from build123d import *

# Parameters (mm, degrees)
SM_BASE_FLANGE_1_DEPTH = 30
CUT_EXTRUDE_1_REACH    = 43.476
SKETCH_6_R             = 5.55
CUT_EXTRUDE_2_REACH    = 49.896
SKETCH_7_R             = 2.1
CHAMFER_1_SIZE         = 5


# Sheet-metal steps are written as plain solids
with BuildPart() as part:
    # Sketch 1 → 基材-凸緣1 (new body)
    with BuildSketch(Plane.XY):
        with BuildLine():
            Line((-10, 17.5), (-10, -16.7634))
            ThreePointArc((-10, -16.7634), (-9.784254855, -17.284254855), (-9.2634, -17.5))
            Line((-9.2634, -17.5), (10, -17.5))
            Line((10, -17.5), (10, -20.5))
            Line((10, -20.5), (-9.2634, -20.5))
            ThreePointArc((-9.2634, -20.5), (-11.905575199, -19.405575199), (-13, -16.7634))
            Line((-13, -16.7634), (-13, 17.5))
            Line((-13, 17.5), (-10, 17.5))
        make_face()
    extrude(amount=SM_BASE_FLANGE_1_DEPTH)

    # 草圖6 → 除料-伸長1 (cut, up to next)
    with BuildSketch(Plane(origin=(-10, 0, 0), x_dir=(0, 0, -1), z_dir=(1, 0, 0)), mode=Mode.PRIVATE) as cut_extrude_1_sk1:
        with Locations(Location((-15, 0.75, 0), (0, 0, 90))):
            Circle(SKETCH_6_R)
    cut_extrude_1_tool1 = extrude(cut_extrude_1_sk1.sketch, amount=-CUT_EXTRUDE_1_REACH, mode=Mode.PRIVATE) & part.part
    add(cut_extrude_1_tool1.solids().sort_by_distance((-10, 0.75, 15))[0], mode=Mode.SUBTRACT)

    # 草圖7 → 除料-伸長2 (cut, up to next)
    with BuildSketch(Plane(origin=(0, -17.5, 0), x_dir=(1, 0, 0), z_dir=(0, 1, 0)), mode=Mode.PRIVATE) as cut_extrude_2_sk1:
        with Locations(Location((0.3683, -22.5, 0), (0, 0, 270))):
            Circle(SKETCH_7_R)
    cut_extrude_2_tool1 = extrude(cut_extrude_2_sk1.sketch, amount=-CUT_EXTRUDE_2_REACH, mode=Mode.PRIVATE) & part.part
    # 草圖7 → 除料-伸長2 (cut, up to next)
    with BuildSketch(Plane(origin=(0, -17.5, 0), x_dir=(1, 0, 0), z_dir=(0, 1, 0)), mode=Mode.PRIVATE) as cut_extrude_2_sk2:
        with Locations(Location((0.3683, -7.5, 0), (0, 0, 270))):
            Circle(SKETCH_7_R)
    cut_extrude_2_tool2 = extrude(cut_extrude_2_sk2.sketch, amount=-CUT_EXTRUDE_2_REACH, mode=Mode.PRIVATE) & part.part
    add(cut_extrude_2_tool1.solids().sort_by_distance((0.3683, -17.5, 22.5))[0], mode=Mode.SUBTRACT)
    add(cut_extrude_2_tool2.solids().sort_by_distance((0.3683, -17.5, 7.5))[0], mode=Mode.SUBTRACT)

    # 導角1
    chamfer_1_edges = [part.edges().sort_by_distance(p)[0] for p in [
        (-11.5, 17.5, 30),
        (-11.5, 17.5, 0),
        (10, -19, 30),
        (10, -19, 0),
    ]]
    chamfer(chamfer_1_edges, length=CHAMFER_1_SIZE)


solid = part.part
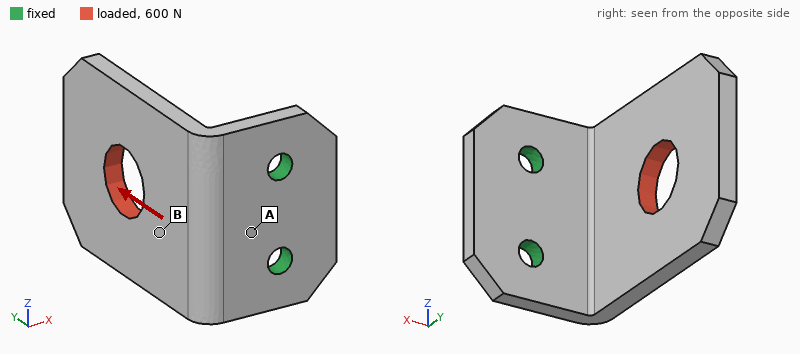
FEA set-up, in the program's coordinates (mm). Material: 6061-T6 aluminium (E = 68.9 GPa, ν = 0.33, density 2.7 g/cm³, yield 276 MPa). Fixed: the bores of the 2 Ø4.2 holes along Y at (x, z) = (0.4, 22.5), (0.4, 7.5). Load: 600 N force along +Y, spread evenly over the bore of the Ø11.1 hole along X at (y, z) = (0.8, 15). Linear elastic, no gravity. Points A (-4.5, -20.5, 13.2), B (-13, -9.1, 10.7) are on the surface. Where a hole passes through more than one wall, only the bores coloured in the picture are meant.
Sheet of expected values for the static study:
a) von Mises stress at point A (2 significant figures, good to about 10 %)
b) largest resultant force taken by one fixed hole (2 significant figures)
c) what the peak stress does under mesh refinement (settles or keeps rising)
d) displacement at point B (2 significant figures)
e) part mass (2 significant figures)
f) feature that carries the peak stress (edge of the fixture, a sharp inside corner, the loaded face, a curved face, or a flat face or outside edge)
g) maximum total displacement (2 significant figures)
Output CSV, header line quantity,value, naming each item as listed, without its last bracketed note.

quantity,value
von Mises stress at point A,73 MPa
largest resultant force taken by one fixed hole,300 N
what the peak stress does under mesh refinement,keeps rising
displacement at point B,0.10 mm
part mass,12 g
feature that carries the peak stress,edge of the fixture
maximum total displacement,0.29 mm
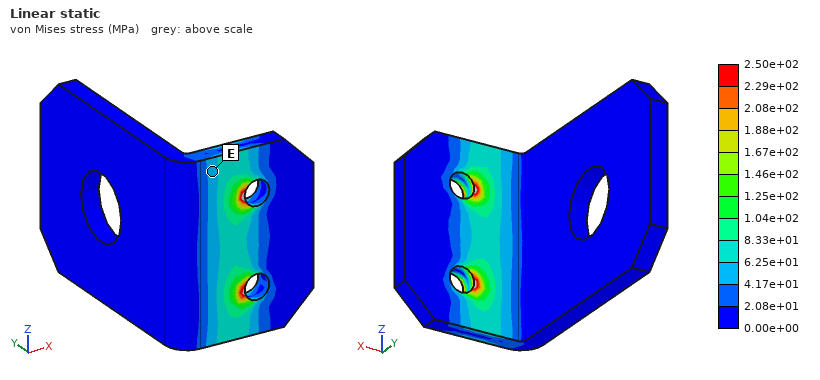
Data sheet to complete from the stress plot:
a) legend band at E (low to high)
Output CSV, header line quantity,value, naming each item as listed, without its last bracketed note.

quantity,value
legend band at E,4.17e+01 to 6.25e+01 MPa
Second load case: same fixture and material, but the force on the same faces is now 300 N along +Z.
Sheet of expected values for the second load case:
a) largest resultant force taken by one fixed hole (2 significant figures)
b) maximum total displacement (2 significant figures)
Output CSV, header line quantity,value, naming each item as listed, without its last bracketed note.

quantity,value
largest resultant force taken by one fixed hole,390 N
maximum total displacement,0.14 mm
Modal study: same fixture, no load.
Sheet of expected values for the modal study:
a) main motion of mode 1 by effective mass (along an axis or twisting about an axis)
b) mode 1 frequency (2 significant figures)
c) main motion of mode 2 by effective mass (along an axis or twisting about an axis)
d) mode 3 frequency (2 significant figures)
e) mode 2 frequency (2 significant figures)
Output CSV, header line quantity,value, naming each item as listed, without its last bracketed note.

quantity,value
main motion of mode 1 by effective mass,along X
mode 1 frequency,1400 Hz
main motion of mode 2 by effective mass,along Z
mode 3 frequency,5000 Hz
mode 2 frequency,3100 Hz
